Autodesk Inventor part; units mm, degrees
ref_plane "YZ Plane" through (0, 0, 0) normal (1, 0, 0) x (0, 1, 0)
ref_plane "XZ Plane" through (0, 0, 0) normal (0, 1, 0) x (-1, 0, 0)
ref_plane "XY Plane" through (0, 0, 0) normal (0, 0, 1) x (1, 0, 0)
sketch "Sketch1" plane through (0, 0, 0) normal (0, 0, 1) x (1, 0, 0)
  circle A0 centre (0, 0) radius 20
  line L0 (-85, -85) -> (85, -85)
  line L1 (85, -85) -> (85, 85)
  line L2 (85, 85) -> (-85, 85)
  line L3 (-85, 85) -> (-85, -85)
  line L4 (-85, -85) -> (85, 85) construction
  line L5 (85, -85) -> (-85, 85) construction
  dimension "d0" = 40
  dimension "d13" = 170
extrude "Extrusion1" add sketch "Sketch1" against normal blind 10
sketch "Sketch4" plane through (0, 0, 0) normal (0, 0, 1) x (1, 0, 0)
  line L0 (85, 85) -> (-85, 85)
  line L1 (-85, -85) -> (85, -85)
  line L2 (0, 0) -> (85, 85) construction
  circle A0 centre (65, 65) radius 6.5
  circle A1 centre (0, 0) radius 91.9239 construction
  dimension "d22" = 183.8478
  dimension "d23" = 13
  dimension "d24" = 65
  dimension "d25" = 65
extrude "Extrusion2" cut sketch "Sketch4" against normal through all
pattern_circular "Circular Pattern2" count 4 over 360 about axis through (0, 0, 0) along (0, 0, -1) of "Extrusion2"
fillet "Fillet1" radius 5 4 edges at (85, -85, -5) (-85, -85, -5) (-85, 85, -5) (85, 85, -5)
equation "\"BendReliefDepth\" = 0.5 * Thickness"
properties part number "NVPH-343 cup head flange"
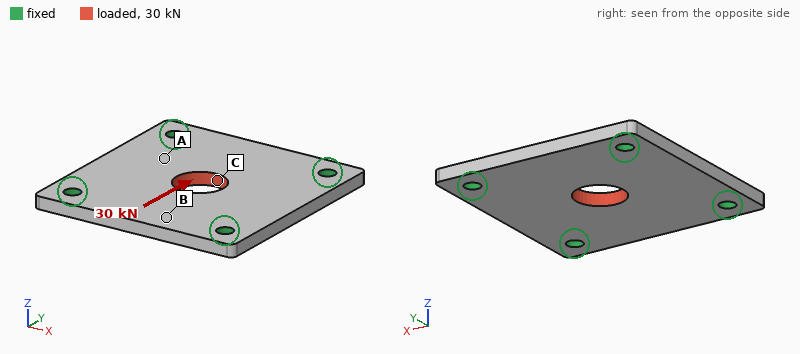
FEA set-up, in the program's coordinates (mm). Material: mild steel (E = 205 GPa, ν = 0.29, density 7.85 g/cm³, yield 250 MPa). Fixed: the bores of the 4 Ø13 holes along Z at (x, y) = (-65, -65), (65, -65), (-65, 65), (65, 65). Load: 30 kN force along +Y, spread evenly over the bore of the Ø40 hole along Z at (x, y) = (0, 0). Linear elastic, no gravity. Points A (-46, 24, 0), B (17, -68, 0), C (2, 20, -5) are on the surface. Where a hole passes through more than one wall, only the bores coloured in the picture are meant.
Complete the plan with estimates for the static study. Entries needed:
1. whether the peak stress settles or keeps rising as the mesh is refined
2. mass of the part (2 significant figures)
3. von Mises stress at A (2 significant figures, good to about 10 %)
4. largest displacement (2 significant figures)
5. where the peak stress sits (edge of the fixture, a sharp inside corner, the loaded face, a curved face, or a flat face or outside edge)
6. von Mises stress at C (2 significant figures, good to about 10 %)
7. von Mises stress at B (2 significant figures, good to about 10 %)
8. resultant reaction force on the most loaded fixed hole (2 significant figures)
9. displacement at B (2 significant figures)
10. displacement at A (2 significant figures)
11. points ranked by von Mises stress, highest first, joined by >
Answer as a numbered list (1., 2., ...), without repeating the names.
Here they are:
1. keeps rising
2. 2.1 kg
3. 16 MPa
4. 9.8 µm
5. edge of the fixture
6. 21 MPa
7. 7.7 MPa
8. 8.3 kN
9. 6.4 µm
10. 4.0 µm
11. C > A > B
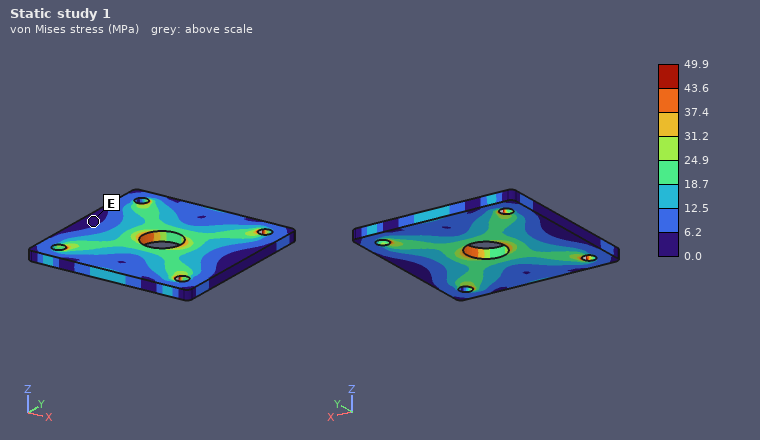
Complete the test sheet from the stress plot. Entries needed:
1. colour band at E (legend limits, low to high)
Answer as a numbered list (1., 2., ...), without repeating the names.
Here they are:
1. 0.0 to 6.2 MPa
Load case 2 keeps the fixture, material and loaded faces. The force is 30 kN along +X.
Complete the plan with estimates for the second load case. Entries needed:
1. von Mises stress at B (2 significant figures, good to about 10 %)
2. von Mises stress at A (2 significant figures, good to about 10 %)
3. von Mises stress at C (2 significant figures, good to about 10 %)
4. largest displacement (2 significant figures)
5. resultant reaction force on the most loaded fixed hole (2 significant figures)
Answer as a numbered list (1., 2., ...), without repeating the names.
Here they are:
1. 6.8 MPa
2. 16 MPa
3. 41 MPa
4. 9.8 µm
5. 8.3 kN
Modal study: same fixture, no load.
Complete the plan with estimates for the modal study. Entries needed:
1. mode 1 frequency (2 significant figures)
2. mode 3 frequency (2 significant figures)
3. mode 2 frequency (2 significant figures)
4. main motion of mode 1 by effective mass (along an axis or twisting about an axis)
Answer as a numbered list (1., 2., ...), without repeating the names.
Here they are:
1. 2300 Hz
2. 3500 Hz
3. 3500 Hz
4. along Z
